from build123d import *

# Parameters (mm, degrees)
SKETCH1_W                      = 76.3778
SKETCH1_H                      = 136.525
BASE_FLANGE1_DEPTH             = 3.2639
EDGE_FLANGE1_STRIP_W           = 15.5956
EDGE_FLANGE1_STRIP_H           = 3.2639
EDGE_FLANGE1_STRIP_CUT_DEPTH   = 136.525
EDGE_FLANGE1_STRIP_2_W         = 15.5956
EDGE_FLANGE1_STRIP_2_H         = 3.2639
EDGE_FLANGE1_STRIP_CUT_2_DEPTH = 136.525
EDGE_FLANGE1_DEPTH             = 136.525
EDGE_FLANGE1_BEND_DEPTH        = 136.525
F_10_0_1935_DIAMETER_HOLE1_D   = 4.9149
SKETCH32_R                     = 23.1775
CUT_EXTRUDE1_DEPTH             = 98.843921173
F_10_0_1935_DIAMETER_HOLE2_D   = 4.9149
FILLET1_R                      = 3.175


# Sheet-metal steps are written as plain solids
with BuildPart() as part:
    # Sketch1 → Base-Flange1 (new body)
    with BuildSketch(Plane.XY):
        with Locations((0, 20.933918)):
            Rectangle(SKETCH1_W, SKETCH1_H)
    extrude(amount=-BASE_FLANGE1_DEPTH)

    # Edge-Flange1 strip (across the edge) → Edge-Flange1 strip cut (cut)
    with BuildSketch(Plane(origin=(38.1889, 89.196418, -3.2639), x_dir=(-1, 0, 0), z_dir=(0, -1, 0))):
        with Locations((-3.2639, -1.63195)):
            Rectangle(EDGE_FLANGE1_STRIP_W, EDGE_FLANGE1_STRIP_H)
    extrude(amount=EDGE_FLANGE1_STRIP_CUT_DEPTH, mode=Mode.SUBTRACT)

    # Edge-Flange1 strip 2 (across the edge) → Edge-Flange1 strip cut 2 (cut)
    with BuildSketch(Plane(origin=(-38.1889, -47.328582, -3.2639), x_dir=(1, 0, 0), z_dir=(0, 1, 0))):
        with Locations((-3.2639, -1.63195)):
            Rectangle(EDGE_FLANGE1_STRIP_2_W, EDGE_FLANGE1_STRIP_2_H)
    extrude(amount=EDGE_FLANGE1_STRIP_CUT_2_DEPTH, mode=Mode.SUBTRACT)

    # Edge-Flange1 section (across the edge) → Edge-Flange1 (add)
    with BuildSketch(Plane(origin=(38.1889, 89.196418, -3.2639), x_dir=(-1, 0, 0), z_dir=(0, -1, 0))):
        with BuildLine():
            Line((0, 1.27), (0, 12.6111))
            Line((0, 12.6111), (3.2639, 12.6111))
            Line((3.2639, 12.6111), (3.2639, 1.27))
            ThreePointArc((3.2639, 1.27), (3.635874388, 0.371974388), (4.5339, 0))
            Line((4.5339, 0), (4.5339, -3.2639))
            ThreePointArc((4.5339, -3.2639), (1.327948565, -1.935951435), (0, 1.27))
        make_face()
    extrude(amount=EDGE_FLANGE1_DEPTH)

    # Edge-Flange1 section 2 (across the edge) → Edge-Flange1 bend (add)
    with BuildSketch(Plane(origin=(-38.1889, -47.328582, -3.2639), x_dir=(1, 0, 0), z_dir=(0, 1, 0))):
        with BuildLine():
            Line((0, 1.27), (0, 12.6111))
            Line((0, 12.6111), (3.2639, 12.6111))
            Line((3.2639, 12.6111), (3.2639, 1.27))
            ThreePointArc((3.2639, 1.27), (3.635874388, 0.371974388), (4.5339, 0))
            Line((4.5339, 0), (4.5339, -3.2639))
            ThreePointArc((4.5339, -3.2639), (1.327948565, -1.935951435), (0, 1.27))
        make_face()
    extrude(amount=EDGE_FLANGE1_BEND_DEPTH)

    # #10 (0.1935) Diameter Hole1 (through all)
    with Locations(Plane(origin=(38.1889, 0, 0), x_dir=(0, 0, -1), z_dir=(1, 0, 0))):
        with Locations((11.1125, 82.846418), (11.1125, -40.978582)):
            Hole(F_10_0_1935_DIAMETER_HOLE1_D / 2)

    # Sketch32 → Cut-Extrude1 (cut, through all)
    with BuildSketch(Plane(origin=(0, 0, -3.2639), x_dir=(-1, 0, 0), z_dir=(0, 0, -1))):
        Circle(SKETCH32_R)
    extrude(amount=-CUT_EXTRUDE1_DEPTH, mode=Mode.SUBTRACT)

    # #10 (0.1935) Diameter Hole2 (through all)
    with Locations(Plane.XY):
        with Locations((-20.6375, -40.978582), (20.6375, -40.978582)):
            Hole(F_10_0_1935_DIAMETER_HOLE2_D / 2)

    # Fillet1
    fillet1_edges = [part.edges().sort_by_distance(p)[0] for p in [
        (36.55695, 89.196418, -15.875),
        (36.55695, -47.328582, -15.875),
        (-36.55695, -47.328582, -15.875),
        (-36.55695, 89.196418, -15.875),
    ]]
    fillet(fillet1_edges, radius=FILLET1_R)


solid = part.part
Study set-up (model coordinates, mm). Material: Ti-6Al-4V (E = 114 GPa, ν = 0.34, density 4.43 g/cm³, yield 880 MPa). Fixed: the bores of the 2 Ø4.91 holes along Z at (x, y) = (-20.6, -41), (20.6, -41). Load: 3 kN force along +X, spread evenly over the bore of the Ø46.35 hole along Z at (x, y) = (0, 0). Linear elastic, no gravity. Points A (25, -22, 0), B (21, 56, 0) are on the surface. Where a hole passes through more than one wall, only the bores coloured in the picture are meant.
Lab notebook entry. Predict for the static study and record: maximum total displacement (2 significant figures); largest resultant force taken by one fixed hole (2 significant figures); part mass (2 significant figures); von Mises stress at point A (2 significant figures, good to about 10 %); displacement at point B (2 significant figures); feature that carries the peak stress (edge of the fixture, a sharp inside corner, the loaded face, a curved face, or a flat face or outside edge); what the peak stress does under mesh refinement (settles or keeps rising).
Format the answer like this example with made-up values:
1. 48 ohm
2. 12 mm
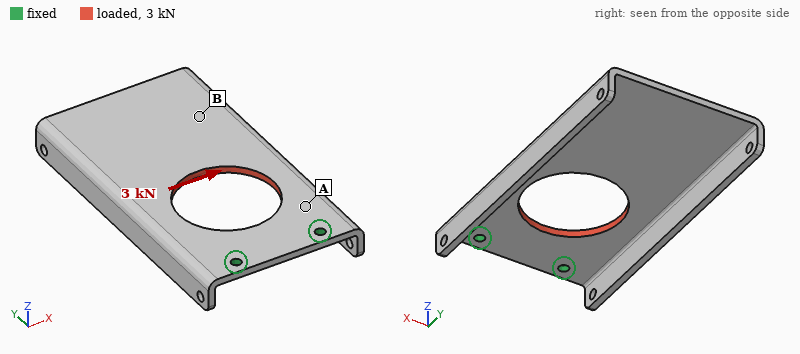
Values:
1. 0.16 mm
2. 3.0 kN
3. 170 g
4. 27 MPa
5. 0.13 mm
6. edge of the fixture
7. keeps rising
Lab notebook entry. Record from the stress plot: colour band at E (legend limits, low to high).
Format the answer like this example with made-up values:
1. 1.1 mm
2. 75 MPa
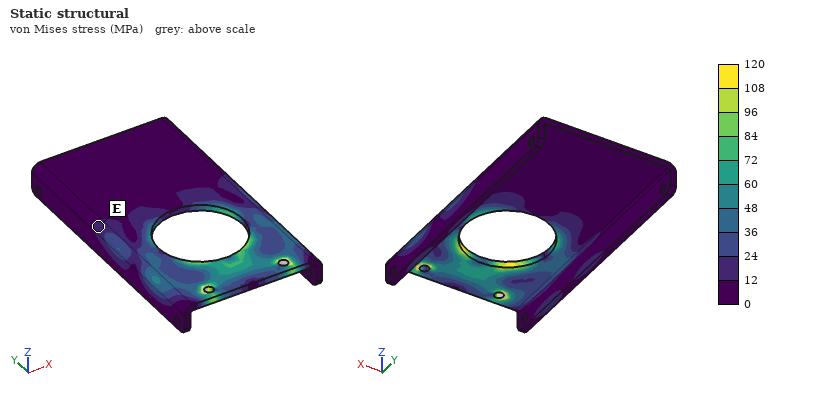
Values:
1. 12 to 24 MPa
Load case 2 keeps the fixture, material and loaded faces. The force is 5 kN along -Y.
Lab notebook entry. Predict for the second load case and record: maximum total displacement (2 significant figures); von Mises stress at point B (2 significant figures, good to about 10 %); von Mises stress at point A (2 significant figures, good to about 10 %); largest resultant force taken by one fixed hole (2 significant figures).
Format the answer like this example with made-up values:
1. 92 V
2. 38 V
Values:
1. 83 µm
2. 5.7 MPa
3. 39 MPa
4. 2.5 kN
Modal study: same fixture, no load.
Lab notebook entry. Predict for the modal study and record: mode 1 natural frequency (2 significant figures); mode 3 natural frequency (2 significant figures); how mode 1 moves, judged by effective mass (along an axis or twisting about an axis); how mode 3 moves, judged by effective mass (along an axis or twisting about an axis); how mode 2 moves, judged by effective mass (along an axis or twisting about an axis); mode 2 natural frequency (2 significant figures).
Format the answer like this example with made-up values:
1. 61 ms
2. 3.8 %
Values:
1. 220 Hz
2. 1500 Hz
3. along Z
4. along X
5. twisting about Y
6. 460 Hz
